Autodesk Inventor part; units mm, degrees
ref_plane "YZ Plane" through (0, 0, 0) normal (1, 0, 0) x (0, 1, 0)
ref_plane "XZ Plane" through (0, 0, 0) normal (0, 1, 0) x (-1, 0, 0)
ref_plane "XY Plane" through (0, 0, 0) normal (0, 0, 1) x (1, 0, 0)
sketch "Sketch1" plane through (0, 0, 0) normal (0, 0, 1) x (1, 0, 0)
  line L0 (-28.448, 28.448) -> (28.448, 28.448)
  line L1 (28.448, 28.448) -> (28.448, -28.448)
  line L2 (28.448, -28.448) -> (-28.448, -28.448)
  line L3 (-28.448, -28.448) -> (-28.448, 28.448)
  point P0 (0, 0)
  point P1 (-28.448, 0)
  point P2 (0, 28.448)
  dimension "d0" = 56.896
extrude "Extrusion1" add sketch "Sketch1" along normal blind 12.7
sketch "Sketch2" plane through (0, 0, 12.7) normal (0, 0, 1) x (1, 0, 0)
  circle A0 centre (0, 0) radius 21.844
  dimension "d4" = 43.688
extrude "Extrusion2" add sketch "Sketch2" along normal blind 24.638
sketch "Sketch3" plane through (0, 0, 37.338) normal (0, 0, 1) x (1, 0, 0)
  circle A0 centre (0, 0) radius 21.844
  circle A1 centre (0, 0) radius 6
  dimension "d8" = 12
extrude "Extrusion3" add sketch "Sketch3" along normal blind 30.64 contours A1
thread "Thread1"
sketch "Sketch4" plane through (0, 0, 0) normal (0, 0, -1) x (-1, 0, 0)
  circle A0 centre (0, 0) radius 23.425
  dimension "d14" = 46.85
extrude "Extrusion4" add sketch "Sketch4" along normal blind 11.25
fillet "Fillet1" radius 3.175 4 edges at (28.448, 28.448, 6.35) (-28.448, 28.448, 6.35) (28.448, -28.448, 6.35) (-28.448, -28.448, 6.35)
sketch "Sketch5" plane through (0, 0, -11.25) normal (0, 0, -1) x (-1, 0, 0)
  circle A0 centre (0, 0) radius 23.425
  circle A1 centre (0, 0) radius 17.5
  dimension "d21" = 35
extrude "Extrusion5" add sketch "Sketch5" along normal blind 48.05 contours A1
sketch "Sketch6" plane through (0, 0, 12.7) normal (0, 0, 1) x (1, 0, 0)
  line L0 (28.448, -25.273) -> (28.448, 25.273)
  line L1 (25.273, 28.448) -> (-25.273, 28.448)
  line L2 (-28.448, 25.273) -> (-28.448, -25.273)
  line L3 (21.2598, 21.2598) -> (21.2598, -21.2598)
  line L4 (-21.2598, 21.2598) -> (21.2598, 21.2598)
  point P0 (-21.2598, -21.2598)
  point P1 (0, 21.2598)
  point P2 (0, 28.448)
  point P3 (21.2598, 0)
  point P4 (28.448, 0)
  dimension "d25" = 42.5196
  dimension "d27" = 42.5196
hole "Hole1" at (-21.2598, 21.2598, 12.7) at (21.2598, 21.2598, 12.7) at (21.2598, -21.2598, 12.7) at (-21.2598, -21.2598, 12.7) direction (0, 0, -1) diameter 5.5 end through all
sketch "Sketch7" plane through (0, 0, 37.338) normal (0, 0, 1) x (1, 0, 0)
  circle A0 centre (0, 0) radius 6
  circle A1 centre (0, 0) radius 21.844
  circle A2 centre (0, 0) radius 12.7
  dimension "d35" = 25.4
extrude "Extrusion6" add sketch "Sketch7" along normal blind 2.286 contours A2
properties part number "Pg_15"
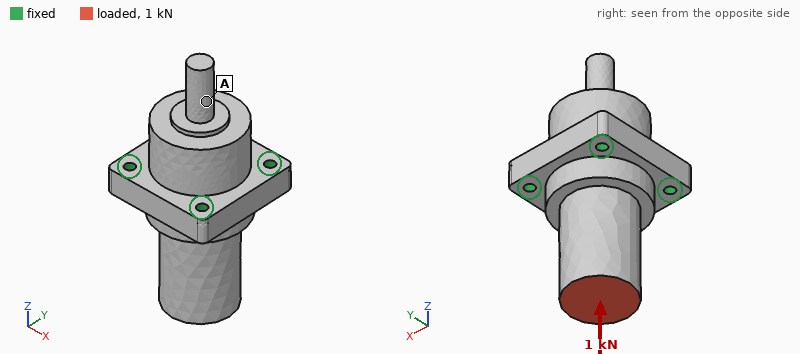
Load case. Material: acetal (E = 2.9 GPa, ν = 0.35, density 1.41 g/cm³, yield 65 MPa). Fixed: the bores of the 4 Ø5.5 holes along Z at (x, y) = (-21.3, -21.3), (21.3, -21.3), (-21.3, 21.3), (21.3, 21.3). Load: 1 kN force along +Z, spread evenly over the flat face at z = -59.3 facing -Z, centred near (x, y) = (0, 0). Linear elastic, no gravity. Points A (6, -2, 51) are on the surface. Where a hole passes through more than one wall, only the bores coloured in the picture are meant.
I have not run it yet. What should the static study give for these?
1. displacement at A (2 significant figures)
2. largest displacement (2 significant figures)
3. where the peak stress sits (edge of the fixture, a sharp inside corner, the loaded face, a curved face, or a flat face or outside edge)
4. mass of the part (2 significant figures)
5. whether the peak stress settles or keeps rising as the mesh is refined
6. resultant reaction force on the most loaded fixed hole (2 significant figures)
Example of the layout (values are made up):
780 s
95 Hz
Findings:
11 µm
33 µm
edge of the fixture
210 g
keeps rising
250 N
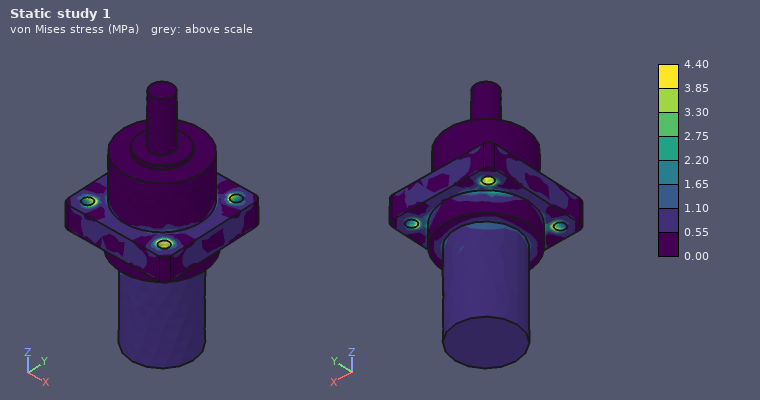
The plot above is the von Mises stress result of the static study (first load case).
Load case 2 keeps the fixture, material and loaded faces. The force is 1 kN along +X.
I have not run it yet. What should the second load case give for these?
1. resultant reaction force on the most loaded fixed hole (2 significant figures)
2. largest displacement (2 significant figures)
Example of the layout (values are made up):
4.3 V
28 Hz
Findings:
850 N
0.48 mm
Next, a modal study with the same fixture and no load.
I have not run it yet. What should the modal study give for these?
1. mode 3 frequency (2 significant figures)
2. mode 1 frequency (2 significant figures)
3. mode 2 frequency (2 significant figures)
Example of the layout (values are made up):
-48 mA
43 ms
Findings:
2200 Hz
1500 Hz
1500 Hz
